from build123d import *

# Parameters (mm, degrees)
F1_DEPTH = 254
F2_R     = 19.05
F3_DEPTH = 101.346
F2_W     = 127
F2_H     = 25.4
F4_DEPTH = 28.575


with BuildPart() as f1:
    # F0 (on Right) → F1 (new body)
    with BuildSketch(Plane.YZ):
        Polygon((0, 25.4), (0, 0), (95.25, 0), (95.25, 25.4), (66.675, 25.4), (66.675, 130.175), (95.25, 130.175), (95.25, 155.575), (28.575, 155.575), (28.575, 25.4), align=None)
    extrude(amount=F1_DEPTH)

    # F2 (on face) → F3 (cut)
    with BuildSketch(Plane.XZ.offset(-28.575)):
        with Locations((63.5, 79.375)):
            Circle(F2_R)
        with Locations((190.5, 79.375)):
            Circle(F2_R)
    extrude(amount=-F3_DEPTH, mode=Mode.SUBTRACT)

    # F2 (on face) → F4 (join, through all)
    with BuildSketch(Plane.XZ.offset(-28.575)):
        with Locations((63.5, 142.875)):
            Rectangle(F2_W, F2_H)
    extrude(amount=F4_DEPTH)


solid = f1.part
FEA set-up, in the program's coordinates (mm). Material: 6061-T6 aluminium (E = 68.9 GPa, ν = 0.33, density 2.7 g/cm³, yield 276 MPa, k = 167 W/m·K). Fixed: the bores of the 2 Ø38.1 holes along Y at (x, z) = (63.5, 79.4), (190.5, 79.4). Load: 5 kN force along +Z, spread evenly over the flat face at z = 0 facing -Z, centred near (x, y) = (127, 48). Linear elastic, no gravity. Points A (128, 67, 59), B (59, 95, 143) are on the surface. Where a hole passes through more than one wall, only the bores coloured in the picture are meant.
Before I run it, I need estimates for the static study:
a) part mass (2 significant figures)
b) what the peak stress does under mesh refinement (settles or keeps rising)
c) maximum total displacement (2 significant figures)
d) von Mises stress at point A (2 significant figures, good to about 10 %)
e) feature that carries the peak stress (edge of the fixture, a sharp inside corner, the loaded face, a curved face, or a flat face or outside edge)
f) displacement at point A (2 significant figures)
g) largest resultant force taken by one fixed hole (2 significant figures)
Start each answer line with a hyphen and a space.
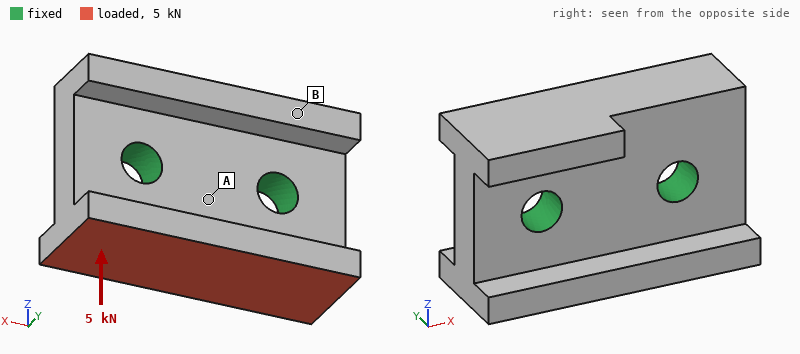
- 5.6 kg
- keeps rising
- 1.4 µm
- 0.24 MPa
- edge of the fixture
- 0.31 µm
- 2.5 kN
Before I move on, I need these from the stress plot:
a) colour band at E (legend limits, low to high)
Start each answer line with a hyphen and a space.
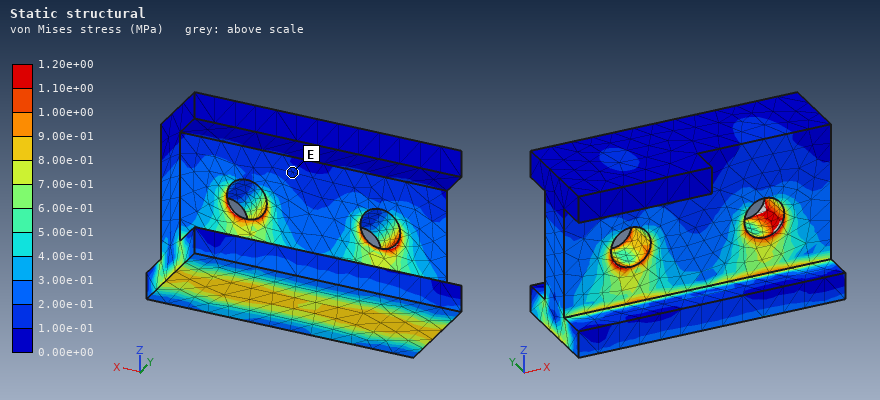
- 1.00e-01 to 2.00e-01 MPa
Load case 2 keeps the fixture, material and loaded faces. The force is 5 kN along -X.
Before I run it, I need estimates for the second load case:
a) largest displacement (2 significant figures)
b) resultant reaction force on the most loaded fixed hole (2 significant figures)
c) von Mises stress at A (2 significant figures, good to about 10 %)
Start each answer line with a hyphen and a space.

- 3.1 µm
- 3.4 kN
- 0.95 MPa
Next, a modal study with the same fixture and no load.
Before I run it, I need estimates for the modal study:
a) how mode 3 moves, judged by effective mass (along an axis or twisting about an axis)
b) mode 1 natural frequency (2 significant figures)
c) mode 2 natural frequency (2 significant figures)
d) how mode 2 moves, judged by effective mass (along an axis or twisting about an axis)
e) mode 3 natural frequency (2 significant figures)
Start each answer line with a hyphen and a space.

- along Y
- 2900 Hz
- 3400 Hz
- along Y
- 3500 Hz
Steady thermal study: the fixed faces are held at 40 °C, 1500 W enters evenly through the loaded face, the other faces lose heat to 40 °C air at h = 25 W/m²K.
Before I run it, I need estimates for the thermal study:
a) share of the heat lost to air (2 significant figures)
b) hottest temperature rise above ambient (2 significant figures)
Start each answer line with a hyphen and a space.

- 5.0 %
- 64 K
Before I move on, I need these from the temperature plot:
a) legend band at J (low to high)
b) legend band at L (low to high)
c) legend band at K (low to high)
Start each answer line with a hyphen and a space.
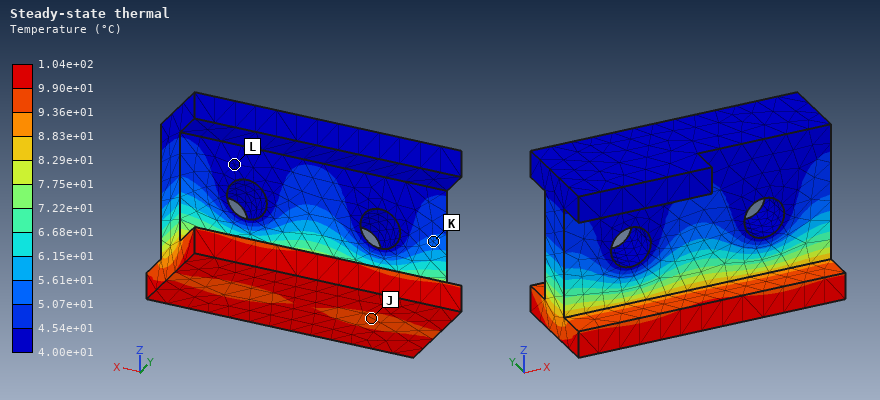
- 9.36e+01 to 9.90e+01 °C
- 4.00e+01 to 4.54e+01 °C
- 5.07e+01 to 5.61e+01 °C
